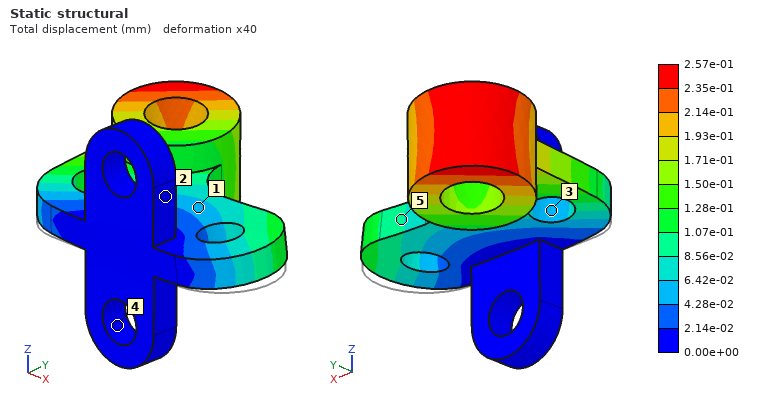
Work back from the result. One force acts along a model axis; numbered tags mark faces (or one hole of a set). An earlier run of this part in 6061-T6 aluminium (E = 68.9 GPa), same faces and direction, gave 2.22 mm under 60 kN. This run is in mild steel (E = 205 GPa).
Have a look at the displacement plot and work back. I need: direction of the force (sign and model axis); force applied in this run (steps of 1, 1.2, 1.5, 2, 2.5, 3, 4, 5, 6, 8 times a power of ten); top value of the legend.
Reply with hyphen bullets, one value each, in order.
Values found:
- +Z
- 20 kN
- 2.57e-01 mm
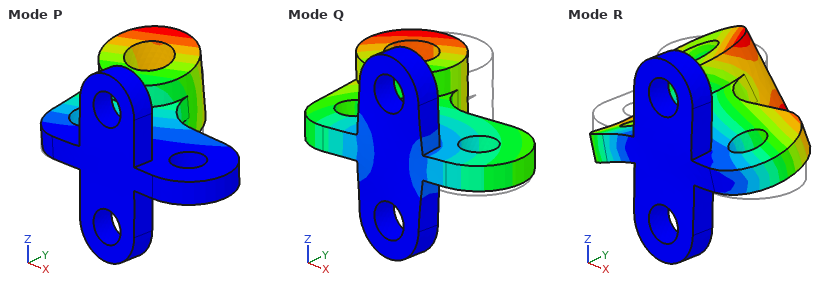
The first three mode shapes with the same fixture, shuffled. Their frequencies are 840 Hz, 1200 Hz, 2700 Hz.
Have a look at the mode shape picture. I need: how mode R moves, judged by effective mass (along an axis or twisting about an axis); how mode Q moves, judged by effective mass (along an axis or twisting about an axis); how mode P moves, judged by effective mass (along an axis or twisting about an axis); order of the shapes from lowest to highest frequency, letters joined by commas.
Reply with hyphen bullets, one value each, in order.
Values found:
- twisting about Y
- along X
- along Z
- P, Q, R
